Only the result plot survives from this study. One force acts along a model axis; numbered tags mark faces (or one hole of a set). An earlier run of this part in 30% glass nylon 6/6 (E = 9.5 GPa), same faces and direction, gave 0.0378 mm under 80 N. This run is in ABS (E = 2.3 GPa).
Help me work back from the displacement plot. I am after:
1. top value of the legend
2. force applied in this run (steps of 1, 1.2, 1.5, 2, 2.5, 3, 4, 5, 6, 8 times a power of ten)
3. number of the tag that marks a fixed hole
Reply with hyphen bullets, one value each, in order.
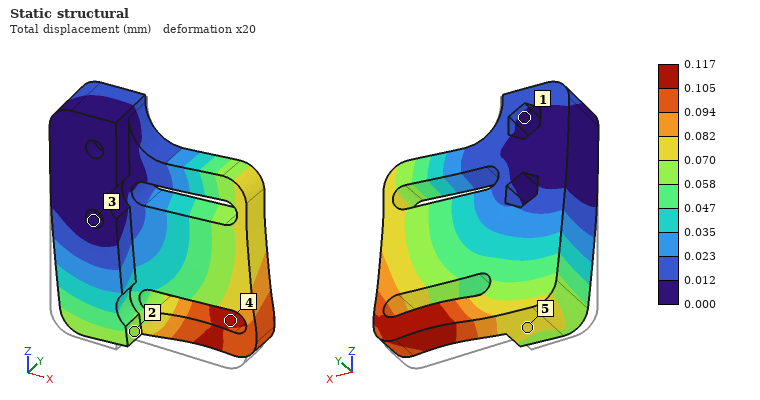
- 0.117 mm
- 60 N
- 3
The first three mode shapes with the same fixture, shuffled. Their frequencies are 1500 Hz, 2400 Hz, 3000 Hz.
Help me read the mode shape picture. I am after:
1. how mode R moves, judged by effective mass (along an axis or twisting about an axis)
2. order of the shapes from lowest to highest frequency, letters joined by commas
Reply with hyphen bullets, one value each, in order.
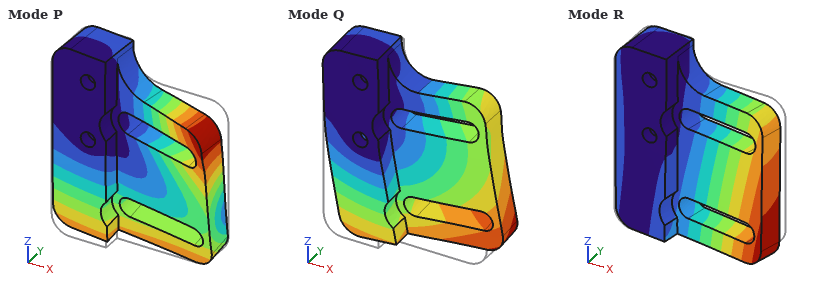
- along Y
- R, Q, P
